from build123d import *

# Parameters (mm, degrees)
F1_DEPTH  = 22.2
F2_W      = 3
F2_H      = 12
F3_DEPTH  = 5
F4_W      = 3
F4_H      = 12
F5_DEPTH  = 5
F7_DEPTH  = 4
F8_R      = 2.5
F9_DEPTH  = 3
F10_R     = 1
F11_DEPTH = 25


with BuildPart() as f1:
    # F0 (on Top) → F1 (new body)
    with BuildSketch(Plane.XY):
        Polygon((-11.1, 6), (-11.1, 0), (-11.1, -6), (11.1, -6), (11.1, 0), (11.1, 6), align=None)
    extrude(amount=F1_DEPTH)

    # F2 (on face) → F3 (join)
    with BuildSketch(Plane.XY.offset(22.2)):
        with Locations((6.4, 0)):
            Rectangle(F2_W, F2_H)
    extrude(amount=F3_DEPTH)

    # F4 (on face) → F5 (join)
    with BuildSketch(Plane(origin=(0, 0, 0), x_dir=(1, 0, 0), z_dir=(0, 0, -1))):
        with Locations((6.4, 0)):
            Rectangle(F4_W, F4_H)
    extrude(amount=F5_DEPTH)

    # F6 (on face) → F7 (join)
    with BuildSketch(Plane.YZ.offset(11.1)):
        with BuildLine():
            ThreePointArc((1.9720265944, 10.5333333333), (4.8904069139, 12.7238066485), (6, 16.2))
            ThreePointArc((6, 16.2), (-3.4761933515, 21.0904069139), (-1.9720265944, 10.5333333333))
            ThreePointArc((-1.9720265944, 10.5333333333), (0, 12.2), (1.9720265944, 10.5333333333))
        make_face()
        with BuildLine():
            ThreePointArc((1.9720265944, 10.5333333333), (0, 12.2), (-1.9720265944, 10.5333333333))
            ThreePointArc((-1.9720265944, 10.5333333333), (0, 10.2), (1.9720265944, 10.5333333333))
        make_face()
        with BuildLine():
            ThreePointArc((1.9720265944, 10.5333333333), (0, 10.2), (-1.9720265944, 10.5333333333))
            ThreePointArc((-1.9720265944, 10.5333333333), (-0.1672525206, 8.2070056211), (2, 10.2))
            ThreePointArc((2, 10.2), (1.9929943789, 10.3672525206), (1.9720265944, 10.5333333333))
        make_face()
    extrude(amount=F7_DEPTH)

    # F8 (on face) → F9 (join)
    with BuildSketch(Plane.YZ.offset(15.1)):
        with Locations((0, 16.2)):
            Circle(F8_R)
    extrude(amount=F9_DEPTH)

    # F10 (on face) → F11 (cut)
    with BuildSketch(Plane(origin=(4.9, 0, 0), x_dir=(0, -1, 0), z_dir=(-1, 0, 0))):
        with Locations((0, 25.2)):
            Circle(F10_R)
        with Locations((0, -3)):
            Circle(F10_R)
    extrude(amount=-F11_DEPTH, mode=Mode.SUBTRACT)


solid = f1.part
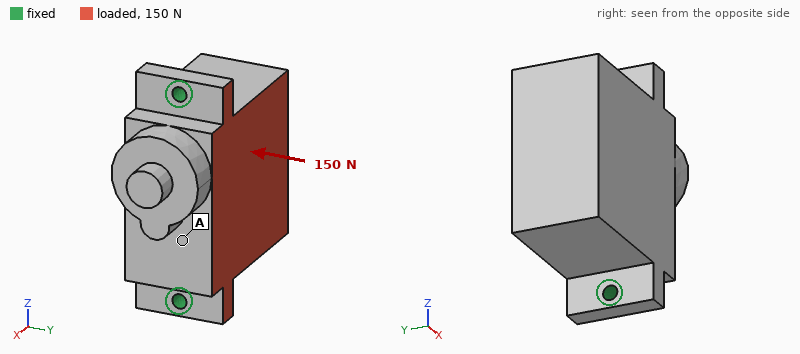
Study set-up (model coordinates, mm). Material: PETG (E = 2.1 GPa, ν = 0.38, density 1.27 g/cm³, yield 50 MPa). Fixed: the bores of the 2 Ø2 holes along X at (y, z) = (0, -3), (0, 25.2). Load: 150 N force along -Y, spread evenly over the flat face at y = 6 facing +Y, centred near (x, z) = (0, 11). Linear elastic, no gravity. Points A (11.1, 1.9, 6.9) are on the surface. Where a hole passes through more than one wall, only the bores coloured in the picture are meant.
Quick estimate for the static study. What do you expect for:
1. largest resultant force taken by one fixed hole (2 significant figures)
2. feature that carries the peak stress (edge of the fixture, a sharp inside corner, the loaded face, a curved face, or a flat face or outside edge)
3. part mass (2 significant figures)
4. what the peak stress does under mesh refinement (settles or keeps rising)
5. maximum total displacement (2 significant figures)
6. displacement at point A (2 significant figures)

75 N
edge of the fixture
8.6 g
keeps rising
0.48 mm
0.093 mm
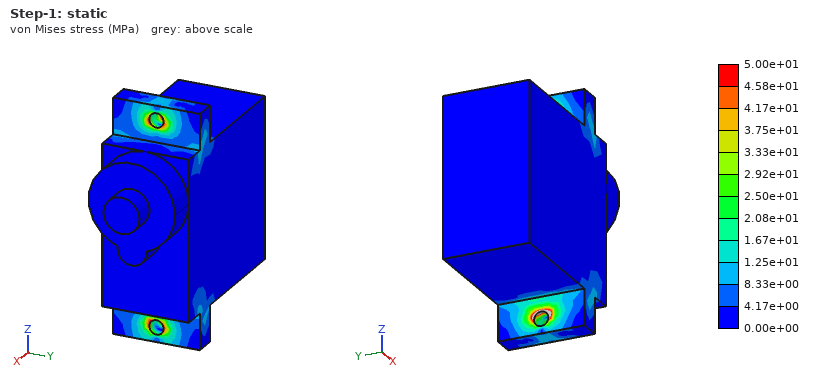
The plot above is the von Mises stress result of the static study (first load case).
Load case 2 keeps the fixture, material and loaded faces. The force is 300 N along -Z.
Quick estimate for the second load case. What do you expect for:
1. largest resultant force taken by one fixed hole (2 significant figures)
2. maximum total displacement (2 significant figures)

180 N
91 µm
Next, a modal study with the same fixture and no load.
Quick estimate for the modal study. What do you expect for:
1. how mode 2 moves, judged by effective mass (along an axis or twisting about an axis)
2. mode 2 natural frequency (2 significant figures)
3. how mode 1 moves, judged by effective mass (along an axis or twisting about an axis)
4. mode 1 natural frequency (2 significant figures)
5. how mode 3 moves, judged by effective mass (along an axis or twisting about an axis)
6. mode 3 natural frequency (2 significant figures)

along X
3900 Hz
along Y
1100 Hz
along Z
4200 Hz
